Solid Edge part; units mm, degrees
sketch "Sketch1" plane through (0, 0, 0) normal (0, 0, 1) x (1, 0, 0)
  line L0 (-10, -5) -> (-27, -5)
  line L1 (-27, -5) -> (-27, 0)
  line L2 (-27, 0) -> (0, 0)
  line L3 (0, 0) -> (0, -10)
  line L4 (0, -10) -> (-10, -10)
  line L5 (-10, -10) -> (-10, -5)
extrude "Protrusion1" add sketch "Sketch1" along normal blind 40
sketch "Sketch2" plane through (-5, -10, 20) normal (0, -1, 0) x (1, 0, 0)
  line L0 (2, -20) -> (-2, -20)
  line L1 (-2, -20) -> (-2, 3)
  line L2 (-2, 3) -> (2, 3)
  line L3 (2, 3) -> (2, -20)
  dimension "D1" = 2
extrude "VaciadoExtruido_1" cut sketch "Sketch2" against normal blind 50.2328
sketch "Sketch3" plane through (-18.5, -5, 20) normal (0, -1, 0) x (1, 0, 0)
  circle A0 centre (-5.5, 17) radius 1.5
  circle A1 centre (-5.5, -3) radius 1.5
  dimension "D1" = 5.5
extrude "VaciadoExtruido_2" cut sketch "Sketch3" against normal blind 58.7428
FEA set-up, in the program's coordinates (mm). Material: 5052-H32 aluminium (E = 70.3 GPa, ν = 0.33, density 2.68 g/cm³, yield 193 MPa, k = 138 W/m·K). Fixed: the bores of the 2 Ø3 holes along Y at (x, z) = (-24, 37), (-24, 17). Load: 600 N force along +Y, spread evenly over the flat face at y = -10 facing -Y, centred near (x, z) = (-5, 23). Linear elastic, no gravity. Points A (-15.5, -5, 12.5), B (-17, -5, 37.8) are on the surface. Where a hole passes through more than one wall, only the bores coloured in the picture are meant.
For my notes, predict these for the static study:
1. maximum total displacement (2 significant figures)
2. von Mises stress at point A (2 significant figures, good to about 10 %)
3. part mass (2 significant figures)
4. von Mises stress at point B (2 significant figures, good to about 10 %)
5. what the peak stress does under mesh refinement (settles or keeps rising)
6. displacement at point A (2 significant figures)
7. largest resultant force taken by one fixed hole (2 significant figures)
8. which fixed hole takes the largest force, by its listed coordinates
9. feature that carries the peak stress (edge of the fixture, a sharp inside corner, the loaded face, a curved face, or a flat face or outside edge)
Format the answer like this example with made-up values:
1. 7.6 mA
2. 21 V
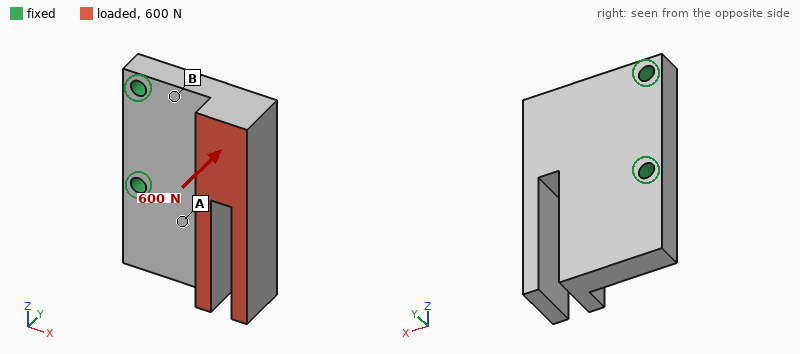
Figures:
1. 0.15 mm
2. 29 MPa
3. 17 g
4. 64 MPa
5. keeps rising
6. 0.025 mm
7. 420 N
8. (-24, 17)
9. edge of the fixture
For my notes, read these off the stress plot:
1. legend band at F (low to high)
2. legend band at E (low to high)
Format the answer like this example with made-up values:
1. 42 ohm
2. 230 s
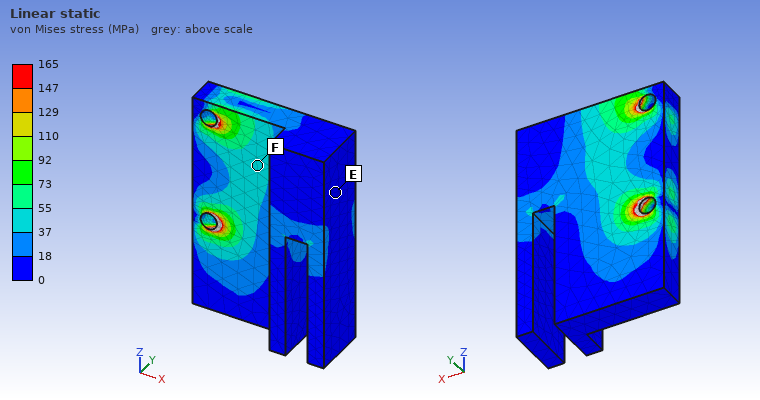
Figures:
1. 37 to 55 MPa
2. 0 to 18 MPa
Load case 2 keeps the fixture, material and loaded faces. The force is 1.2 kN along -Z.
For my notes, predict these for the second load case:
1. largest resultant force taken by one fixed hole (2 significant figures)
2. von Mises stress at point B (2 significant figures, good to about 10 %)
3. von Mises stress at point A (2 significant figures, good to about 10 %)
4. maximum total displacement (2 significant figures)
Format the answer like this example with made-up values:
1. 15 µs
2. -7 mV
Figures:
1. 1.3 kN
2. 40 MPa
3. 22 MPa
4. 89 µm
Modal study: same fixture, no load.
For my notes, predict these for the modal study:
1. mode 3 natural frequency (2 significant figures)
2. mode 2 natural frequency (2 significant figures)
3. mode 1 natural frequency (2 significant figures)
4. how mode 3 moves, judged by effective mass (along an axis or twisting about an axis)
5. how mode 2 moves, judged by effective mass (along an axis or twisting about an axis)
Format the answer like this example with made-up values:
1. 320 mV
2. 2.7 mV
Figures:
1. 7600 Hz
2. 4400 Hz
3. 4000 Hz
4. twisting about X
5. along Y
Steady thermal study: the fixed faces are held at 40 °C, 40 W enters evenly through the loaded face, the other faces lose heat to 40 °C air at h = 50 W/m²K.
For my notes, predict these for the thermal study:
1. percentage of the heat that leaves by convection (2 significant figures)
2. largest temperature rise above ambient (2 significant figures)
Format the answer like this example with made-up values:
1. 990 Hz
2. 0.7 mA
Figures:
1. 10 %
2. 65 K
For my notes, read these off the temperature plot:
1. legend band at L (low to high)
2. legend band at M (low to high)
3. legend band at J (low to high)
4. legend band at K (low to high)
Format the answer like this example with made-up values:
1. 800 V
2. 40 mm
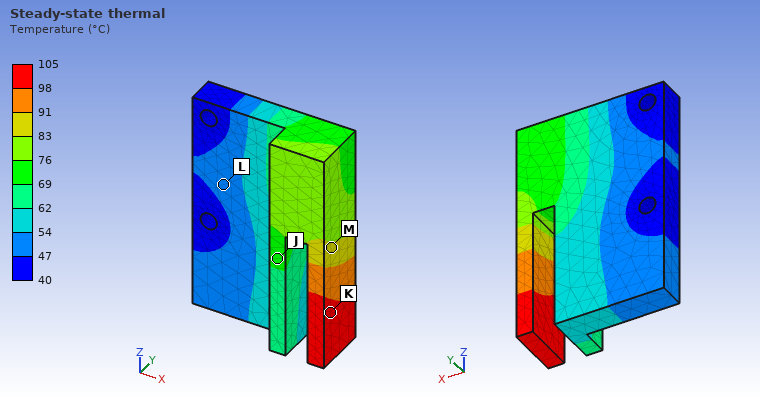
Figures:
1. 47 to 54 °C
2. 83 to 91 °C
3. 69 to 76 °C
4. 98 to 105 °C
